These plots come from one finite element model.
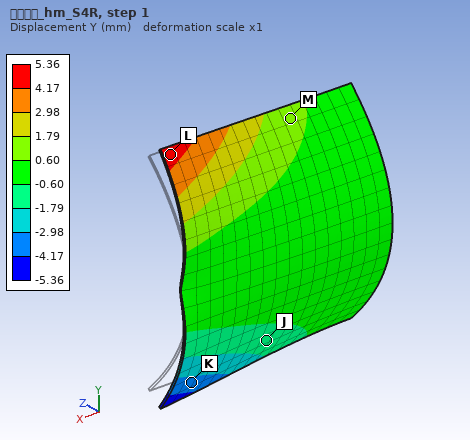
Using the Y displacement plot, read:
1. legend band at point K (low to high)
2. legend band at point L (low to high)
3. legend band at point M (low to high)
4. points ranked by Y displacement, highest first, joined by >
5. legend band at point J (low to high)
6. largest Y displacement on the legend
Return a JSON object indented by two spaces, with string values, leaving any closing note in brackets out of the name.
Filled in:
{
  "legend band at point K": "-4.17 to -2.98 mm",
  "legend band at point L": "4.17 to 5.36 mm",
  "legend band at point M": "0.60 to 1.79 mm",
  "points ranked by Y displacement, highest first, joined by >": "L > M > J > K",
  "legend band at point J": "-1.79 to -0.60 mm",
  "largest Y displacement on the legend": "5.36 mm"
}
